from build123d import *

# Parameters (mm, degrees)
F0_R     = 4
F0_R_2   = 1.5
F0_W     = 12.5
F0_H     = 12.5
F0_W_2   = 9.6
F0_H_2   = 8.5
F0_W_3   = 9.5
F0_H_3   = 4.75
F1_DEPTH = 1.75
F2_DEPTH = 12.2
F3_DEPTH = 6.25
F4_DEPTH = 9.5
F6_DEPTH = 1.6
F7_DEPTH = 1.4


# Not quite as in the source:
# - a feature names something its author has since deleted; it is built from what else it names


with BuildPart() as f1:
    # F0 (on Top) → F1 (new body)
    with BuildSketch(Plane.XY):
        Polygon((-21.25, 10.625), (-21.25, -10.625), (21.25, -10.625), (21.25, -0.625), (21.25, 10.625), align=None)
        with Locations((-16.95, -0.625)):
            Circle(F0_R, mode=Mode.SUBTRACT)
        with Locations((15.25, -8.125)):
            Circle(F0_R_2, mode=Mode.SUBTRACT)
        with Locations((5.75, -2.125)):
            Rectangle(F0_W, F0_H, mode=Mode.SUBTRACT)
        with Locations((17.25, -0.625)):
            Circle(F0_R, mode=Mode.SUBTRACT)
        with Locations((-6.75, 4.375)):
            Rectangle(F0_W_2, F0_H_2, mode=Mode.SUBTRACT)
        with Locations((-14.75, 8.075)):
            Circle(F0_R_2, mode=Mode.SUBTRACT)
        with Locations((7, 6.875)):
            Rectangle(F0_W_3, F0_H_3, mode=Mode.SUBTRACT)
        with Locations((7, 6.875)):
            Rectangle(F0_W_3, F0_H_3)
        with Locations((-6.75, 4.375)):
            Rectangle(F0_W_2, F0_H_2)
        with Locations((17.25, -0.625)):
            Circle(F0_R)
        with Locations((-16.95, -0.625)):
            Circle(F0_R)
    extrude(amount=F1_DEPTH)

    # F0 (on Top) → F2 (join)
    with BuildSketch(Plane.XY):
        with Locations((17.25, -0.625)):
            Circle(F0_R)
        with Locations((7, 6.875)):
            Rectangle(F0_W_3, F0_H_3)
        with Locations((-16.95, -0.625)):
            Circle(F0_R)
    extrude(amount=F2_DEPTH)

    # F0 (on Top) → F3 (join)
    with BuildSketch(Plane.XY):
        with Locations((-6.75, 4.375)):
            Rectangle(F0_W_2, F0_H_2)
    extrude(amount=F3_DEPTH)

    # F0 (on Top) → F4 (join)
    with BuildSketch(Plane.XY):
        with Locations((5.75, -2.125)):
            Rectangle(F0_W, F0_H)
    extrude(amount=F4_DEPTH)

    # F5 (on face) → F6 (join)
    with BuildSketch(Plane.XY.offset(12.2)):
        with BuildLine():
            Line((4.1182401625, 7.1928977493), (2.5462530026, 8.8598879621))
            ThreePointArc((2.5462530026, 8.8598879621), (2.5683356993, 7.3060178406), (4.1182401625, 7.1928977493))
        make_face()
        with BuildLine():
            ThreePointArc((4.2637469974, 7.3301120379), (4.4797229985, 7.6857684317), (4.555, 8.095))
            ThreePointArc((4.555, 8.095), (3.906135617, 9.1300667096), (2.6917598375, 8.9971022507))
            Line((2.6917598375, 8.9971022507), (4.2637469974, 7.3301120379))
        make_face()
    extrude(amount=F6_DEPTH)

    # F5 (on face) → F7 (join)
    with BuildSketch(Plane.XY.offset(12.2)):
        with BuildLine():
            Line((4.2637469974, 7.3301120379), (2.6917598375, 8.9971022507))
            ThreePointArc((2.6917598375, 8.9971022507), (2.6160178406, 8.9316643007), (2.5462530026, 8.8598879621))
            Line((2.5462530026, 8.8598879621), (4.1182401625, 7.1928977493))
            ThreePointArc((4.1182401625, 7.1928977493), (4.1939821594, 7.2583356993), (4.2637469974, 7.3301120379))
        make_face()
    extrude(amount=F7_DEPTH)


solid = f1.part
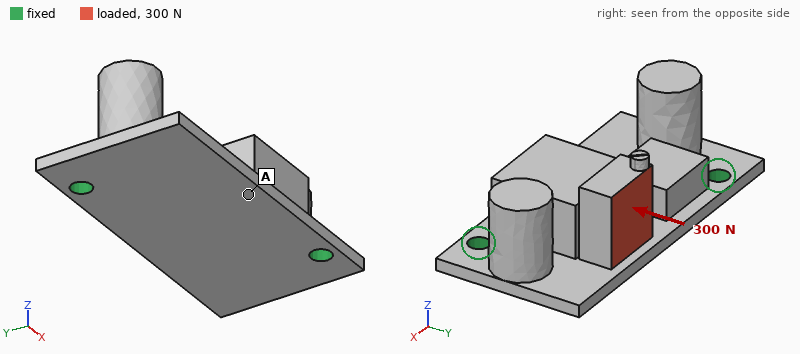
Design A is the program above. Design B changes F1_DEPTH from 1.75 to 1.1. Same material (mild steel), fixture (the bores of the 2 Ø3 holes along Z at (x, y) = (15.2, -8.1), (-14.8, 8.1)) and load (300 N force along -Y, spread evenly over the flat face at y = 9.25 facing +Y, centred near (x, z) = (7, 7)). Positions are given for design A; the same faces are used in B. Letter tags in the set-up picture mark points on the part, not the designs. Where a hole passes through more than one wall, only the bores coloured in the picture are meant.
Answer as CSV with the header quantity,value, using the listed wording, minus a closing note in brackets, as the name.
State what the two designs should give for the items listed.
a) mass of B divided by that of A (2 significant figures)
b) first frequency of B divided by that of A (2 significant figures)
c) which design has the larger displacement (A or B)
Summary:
quantity,value
mass of B divided by that of A,0.93
first frequency of B divided by that of A,0.60
which design has the larger displacement,B
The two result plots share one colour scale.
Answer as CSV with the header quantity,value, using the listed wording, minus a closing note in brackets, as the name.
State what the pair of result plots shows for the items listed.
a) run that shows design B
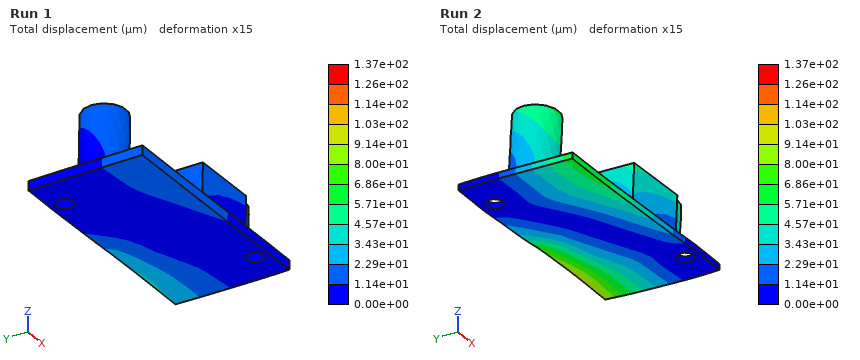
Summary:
quantity,value
run that shows design B,Run 2
